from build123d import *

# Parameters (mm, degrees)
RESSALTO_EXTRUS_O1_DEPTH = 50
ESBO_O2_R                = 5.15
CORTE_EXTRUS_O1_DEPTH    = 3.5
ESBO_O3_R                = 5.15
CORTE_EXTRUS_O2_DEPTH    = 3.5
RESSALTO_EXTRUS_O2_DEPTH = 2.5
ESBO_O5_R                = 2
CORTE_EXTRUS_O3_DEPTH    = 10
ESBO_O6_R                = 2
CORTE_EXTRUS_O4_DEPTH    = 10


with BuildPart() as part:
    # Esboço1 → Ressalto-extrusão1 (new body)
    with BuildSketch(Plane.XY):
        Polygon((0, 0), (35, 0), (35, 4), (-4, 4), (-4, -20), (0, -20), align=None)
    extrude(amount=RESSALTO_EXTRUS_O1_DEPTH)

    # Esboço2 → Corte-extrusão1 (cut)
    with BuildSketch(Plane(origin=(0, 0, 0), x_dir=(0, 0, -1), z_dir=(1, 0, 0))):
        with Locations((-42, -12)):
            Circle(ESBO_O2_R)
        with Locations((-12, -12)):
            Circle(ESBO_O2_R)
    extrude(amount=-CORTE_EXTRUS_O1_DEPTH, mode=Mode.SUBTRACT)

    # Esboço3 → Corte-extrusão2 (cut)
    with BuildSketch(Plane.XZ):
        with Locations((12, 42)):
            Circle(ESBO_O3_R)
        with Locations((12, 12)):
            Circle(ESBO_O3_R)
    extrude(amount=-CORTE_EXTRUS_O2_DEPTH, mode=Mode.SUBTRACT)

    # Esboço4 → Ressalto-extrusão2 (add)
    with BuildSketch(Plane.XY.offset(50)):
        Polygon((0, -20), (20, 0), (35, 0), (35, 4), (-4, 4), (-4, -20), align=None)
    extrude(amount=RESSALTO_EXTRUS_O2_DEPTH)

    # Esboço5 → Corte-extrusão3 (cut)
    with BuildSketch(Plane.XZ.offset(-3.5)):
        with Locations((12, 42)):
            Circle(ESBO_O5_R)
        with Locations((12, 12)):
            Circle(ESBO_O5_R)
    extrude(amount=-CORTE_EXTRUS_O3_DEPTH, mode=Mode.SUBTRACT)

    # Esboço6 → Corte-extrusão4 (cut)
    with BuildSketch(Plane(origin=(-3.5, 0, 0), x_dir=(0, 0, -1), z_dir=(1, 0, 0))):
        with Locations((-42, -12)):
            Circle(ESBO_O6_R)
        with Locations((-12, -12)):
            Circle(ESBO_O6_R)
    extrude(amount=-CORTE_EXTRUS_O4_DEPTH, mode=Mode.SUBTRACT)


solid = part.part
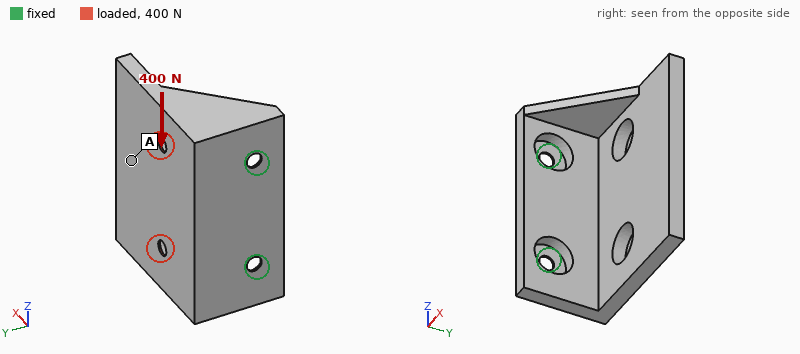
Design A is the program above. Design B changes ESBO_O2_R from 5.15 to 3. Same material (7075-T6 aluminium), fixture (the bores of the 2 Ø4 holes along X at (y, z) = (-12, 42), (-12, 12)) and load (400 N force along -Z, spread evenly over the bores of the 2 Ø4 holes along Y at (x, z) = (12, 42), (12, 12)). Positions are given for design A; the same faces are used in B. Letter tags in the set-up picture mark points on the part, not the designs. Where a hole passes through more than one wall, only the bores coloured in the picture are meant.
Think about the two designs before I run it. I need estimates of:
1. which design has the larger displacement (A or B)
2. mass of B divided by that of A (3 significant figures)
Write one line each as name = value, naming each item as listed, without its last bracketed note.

which design has the larger displacement = A
mass of B divided by that of A = 1.03
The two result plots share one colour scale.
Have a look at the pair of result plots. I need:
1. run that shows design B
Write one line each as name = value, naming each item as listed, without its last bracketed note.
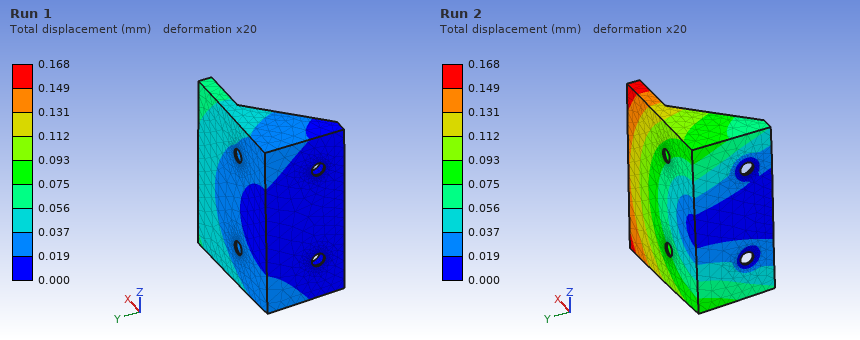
run that shows design B = Run 1
